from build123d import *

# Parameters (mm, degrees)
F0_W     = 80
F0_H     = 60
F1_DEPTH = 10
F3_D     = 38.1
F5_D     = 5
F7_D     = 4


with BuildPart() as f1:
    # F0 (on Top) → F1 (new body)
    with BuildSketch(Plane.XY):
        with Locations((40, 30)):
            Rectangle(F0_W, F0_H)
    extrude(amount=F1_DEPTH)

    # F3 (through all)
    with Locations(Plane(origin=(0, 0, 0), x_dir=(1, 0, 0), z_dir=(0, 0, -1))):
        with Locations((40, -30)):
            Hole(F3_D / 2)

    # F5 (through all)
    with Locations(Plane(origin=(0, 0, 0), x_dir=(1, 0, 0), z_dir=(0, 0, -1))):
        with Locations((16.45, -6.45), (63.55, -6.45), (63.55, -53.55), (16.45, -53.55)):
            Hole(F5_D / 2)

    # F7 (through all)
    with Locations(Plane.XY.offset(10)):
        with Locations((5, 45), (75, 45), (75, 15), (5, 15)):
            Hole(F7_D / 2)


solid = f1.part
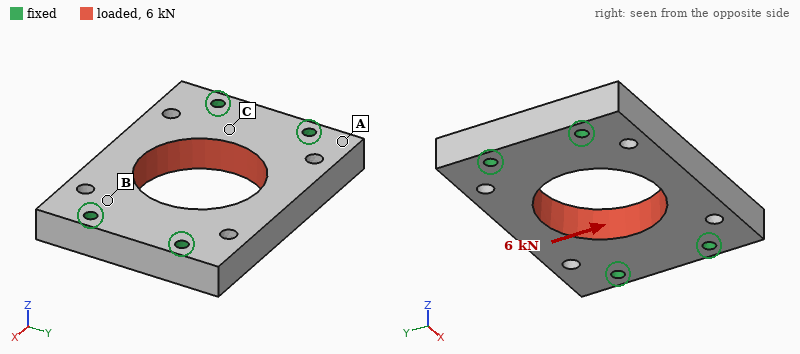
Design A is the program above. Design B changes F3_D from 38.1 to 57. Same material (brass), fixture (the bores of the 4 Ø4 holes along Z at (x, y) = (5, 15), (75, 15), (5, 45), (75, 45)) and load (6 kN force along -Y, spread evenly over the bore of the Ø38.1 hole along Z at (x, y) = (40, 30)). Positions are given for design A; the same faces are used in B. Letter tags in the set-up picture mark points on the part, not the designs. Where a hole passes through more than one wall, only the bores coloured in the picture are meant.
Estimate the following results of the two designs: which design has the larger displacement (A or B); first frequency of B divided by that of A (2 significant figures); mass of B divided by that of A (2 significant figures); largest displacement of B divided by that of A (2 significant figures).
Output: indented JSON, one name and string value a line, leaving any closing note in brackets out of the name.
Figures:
{
  "which design has the larger displacement": "B",
  "first frequency of B divided by that of A": "1.2",
  "mass of B divided by that of A": "0.60",
  "largest displacement of B divided by that of A": "5.4"
}
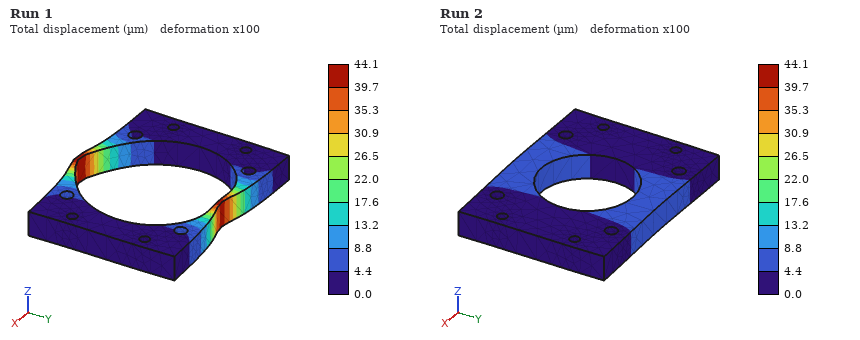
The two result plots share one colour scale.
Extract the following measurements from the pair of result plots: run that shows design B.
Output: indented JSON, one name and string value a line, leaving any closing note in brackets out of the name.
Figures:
{
  "run that shows design B": "Run 1"
}
